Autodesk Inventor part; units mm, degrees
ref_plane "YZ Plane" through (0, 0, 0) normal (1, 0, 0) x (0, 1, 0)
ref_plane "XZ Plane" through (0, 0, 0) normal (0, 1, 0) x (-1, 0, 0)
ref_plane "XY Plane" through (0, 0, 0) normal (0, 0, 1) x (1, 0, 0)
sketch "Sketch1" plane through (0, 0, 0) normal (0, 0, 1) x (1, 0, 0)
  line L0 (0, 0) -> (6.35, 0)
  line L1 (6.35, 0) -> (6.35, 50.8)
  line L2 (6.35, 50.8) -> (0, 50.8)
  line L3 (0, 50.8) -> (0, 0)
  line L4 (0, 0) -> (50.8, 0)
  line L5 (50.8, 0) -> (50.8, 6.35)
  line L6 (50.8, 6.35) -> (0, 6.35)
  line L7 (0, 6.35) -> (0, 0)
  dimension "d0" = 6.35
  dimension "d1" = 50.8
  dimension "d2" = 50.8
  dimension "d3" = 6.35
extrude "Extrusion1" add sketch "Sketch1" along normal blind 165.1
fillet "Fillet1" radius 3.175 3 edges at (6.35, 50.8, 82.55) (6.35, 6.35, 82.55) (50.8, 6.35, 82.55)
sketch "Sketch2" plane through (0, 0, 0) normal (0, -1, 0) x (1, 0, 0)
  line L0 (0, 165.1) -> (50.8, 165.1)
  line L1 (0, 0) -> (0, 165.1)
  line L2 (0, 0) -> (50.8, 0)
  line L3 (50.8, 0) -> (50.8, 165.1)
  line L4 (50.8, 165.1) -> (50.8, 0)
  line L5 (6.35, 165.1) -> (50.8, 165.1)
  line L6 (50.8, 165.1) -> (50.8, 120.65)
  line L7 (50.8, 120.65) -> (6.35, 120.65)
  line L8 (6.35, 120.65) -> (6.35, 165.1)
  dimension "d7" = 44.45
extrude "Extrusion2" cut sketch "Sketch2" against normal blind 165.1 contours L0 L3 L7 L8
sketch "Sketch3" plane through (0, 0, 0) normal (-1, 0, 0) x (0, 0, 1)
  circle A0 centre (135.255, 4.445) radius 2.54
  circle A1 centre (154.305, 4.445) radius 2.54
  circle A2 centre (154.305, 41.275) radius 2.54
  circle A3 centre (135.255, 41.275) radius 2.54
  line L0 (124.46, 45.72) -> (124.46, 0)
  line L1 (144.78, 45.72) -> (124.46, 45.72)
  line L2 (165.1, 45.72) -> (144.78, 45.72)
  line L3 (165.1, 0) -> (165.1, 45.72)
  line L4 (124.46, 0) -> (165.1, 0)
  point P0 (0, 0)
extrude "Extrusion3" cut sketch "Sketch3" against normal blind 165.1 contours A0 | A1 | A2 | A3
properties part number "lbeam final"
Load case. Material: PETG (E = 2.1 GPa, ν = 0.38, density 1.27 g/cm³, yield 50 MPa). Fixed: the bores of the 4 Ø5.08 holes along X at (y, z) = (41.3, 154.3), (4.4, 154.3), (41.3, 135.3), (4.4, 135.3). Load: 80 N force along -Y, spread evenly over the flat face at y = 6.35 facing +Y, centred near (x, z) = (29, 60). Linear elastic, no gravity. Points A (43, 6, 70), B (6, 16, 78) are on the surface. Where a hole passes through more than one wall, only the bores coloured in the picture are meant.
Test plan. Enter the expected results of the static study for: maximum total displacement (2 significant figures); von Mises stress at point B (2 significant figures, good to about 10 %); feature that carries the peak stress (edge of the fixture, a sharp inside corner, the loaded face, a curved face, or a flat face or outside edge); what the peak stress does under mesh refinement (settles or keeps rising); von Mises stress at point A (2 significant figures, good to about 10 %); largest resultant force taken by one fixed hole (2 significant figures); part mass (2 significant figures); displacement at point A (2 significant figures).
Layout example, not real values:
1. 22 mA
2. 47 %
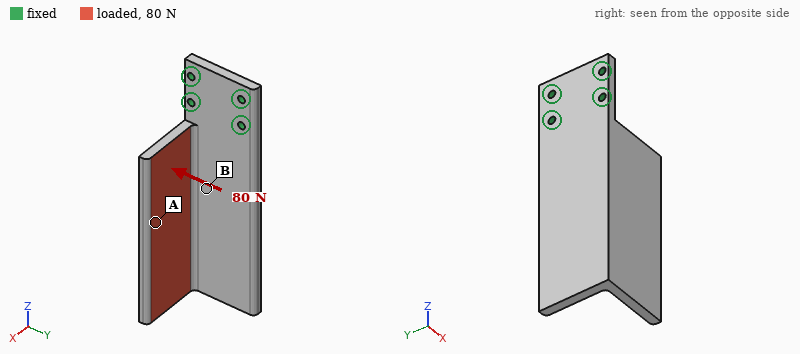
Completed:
1. 2.0 mm
2. 2.9 MPa
3. edge of the fixture
4. keeps rising
5. 0.89 MPa
6. 160 N
7. 110 g
8. 1.1 mm
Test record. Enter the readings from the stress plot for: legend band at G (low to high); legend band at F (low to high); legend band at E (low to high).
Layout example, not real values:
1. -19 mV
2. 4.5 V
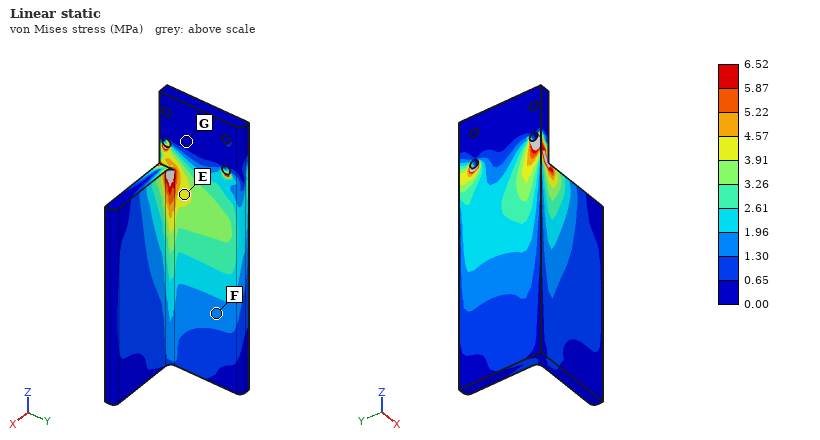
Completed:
1. 0.00 to 0.65 MPa
2. 1.30 to 1.96 MPa
3. 3.91 to 4.57 MPa
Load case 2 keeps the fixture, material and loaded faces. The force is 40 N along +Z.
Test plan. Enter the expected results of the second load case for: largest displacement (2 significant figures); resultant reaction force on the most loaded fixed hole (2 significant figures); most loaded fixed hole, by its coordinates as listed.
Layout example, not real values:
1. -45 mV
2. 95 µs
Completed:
1. 1.7 mm
2. 34 N
3. (4.4, 135.3)
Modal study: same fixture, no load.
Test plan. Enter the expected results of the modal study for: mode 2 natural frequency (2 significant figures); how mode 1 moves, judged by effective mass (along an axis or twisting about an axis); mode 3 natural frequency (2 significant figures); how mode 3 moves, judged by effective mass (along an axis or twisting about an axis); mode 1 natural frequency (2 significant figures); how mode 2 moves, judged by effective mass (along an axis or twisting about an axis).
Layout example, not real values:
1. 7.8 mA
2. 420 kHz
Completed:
1. 200 Hz
2. along X
3. 430 Hz
4. along Y
5. 63 Hz
6. along Y
